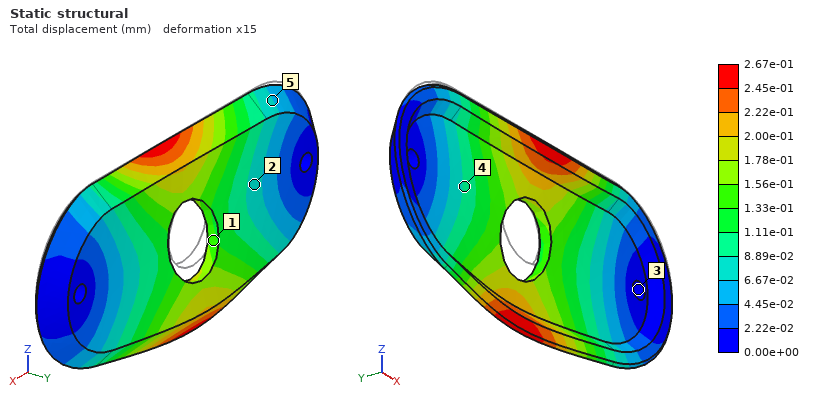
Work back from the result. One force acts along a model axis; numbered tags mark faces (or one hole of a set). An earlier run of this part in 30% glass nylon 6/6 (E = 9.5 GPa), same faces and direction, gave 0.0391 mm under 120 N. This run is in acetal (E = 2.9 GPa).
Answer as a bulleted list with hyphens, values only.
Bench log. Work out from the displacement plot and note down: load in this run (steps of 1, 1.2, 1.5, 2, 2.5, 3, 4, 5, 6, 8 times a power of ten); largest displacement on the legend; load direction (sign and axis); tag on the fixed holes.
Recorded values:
- 250 N
- 2.67e-01 mm
- -Z
- 3
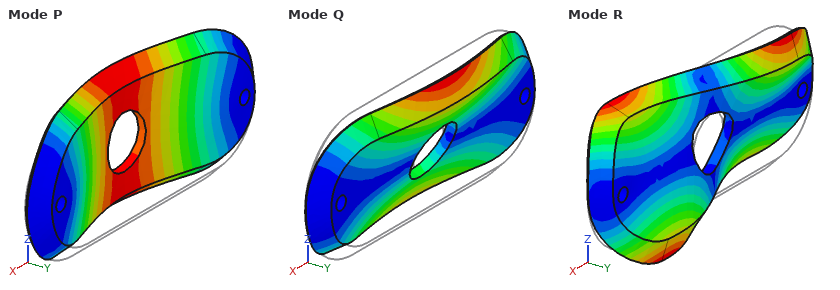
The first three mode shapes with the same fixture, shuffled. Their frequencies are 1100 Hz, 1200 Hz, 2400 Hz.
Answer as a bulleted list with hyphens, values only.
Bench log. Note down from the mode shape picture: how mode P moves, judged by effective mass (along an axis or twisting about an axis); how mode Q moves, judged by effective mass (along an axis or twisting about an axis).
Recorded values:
- along Y
- twisting about X
